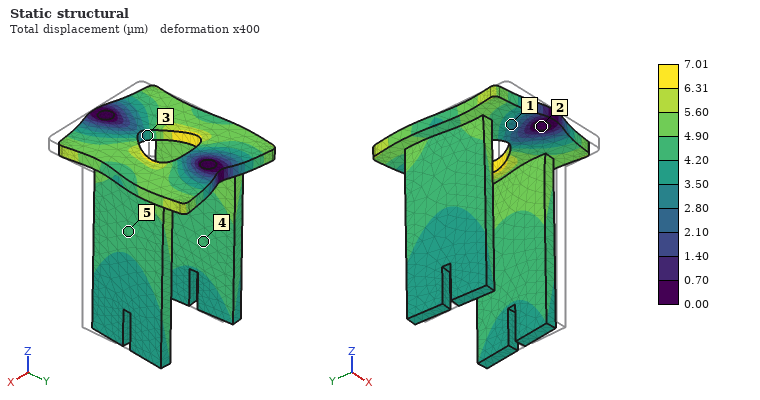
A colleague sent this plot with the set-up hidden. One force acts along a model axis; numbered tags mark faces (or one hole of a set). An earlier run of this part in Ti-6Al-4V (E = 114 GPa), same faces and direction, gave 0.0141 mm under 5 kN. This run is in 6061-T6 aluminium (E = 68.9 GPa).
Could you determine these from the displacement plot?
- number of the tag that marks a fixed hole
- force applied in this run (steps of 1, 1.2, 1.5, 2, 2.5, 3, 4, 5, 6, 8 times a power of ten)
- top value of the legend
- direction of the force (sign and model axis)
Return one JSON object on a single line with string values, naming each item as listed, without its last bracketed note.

{"number of the tag that marks a fixed hole": "2", "force applied in this run": "1.5 kN", "top value of the legend": "7.01 µm", "direction of the force": "+Y"}
